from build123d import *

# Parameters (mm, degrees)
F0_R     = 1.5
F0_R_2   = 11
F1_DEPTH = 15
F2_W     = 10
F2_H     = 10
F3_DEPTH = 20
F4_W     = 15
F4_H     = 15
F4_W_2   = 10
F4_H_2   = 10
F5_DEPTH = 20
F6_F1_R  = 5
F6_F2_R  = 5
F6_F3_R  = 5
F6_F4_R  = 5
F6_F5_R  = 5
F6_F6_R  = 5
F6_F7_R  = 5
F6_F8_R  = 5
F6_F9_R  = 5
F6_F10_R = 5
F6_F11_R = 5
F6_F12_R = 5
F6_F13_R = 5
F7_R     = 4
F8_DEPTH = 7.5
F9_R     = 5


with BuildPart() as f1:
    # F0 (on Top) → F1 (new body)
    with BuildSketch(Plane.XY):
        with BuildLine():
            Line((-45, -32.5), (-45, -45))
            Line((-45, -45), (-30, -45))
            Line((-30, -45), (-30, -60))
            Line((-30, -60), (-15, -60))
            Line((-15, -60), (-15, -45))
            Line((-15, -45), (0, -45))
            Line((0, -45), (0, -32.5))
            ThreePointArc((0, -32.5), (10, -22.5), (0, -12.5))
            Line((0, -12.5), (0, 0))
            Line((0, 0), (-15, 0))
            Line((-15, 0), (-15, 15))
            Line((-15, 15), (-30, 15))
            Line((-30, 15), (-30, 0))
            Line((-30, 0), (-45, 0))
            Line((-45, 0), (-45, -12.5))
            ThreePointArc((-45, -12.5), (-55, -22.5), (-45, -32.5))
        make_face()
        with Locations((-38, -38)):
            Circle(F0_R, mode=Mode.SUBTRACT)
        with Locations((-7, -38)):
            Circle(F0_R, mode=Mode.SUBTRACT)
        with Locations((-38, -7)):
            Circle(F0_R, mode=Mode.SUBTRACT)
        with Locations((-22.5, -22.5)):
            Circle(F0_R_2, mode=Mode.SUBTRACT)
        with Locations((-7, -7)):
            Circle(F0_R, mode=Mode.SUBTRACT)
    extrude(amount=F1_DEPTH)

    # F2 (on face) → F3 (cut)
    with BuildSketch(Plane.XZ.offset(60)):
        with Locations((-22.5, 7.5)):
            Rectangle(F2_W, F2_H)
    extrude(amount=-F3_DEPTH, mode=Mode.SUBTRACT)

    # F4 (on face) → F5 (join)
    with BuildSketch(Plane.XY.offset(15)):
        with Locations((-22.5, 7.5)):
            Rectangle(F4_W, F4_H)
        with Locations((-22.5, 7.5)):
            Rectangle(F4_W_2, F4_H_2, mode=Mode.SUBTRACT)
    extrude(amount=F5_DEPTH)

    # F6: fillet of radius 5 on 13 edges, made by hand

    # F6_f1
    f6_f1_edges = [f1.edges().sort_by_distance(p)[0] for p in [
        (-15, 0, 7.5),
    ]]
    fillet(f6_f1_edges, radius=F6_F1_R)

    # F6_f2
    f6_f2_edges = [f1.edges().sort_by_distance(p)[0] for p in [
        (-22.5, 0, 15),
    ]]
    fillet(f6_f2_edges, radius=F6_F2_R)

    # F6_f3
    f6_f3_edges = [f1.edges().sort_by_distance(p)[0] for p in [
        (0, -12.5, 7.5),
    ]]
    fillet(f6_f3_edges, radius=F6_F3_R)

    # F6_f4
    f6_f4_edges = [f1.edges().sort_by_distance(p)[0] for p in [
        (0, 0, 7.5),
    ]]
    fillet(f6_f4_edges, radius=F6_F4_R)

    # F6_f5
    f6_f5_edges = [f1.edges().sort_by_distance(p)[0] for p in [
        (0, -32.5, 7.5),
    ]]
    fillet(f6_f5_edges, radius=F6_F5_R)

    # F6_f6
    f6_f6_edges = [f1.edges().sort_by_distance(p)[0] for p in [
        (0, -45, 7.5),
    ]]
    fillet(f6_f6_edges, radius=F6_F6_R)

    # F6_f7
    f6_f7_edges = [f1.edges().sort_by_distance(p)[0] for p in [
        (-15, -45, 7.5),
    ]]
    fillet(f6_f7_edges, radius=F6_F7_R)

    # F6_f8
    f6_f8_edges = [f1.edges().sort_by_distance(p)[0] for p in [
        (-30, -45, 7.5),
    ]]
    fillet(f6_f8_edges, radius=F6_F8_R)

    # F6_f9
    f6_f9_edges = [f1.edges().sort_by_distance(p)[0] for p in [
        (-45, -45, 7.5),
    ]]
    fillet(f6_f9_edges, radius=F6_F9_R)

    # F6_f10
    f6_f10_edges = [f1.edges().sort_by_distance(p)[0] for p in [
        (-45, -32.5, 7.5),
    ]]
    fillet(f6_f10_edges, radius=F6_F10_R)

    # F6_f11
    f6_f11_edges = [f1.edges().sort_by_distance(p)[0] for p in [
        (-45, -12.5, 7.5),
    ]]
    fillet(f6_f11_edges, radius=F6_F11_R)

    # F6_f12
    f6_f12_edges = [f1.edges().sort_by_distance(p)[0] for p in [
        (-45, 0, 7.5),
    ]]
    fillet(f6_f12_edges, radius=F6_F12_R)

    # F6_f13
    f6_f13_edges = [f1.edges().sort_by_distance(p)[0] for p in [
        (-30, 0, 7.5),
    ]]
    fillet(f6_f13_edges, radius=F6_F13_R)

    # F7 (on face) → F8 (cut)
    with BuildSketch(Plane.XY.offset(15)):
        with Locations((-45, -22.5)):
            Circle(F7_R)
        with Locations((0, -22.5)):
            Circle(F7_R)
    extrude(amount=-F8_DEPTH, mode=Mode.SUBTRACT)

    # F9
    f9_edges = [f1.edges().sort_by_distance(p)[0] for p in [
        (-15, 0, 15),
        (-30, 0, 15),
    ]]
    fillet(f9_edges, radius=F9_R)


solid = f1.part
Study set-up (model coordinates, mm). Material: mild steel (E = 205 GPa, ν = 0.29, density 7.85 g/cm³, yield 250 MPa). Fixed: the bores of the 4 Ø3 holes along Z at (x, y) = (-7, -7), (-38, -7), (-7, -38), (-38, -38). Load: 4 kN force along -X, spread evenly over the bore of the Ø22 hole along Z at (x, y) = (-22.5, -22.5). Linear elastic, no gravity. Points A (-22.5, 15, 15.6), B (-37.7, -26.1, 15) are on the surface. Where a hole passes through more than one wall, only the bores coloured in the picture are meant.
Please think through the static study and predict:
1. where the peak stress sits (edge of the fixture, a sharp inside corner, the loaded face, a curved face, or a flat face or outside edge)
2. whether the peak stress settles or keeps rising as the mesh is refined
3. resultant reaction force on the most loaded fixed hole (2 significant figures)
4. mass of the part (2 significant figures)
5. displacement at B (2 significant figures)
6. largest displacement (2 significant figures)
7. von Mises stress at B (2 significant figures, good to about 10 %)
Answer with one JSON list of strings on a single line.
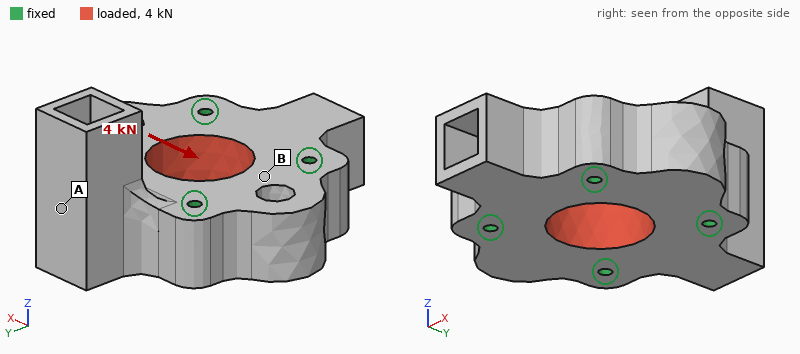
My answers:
["edge of the fixture", "keeps rising", "1.0 kN", "280 g", "0.53 µm", "0.67 µm", "4.6 MPa"]
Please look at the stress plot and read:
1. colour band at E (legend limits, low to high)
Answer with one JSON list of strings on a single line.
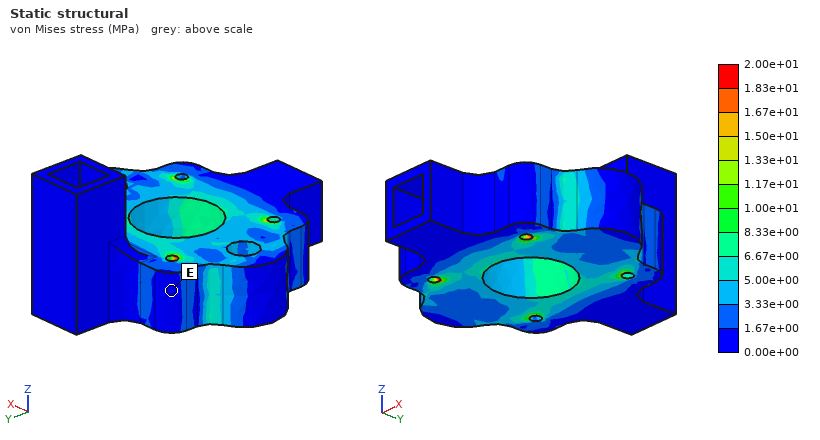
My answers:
["0.00e+00 to 1.67e+00 MPa"]
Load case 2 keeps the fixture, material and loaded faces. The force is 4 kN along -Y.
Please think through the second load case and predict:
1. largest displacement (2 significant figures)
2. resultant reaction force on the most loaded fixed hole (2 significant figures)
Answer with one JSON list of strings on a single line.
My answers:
["0.71 µm", "1.0 kN"]
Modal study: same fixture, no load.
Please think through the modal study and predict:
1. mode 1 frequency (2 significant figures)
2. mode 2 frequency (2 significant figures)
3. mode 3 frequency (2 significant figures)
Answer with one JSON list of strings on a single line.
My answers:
["9500 Hz", "14 kHz", "19 kHz"]
